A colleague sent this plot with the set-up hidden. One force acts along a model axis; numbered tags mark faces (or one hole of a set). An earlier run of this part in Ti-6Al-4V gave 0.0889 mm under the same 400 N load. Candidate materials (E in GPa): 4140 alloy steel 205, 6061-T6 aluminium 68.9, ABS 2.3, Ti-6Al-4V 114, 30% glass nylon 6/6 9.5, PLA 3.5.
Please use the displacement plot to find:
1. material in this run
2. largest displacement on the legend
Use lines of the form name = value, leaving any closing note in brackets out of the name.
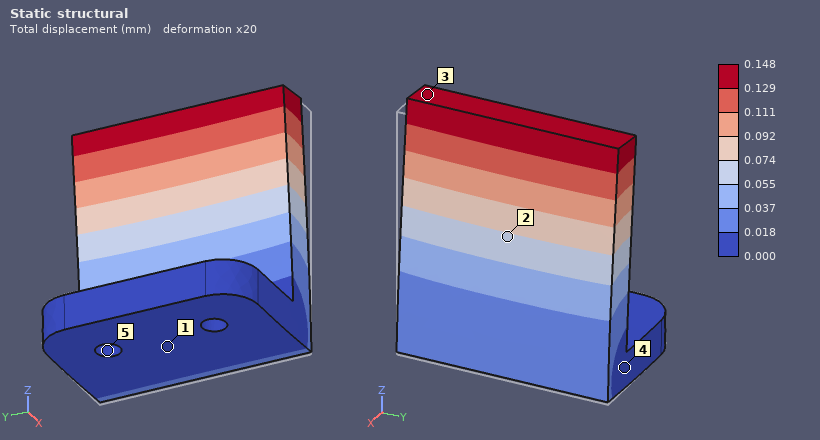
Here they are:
material in this run = 6061-T6 aluminium
largest displacement on the legend = 0.148 mm
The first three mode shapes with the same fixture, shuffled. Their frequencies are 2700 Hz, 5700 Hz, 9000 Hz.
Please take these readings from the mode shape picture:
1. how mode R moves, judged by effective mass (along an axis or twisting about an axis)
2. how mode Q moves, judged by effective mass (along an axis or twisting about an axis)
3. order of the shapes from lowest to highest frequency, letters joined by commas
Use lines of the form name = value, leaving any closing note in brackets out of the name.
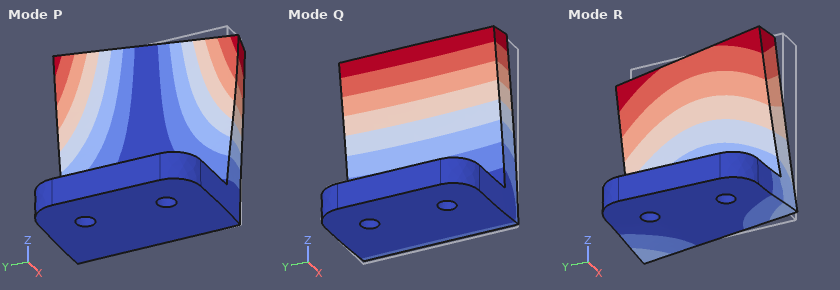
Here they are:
how mode R moves, judged by effective mass = along Y
how mode Q moves, judged by effective mass = along X
order of the shapes from lowest to highest frequency, letters joined by commas = Q, R, P
